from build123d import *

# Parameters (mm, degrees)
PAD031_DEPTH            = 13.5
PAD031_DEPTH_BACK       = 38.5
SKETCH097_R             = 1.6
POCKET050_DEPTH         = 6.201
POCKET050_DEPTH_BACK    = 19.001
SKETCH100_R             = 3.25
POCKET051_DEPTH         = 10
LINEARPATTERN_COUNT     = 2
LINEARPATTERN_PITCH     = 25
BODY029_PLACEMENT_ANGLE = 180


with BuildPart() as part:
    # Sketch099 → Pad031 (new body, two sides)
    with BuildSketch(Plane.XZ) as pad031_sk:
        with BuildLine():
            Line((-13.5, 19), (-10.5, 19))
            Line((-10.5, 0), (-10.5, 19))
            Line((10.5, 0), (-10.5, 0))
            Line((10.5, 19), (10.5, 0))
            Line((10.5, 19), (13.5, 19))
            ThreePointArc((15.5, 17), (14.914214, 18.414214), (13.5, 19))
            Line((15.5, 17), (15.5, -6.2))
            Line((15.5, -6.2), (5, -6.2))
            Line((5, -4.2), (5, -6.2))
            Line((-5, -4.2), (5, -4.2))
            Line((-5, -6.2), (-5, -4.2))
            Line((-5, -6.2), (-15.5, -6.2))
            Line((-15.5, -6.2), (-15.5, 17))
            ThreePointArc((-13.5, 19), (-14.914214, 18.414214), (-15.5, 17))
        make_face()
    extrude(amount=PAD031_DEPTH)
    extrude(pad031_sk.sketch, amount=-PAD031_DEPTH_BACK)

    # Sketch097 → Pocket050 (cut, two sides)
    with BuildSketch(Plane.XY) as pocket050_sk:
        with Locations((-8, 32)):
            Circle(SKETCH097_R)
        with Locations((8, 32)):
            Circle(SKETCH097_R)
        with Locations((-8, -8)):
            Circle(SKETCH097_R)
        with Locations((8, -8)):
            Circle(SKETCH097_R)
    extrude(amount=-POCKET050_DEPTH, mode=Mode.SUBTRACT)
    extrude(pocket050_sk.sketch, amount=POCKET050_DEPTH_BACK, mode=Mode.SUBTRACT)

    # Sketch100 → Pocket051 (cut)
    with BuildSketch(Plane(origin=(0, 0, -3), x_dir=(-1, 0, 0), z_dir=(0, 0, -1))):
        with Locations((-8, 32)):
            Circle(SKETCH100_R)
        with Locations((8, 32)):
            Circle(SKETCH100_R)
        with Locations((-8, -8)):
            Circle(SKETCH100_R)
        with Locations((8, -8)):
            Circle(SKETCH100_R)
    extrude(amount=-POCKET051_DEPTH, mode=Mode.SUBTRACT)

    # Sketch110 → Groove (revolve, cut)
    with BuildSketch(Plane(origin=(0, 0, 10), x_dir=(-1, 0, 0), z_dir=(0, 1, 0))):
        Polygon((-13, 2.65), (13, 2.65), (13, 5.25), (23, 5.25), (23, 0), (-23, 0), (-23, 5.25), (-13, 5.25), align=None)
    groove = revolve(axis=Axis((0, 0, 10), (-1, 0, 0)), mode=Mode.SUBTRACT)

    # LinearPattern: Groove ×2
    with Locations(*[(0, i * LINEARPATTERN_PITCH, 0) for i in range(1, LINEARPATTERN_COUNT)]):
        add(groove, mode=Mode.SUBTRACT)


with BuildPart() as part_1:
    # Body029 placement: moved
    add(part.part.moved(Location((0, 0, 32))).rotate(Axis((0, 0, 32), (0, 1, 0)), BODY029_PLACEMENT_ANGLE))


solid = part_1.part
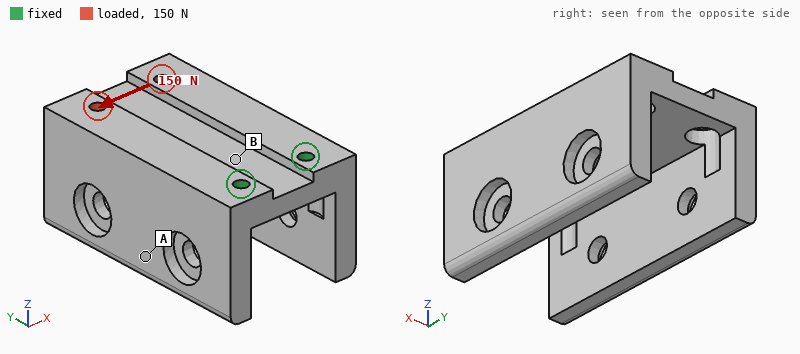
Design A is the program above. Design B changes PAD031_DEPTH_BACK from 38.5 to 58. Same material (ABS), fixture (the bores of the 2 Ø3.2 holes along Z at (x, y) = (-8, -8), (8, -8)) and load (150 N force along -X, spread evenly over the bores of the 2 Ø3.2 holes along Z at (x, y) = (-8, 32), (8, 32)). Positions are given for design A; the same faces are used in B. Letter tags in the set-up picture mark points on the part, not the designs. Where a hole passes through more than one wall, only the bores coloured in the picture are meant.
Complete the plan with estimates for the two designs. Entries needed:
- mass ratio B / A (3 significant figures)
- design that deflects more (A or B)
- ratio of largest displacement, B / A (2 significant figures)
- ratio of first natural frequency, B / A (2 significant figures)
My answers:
1.41
B
1.2
0.59
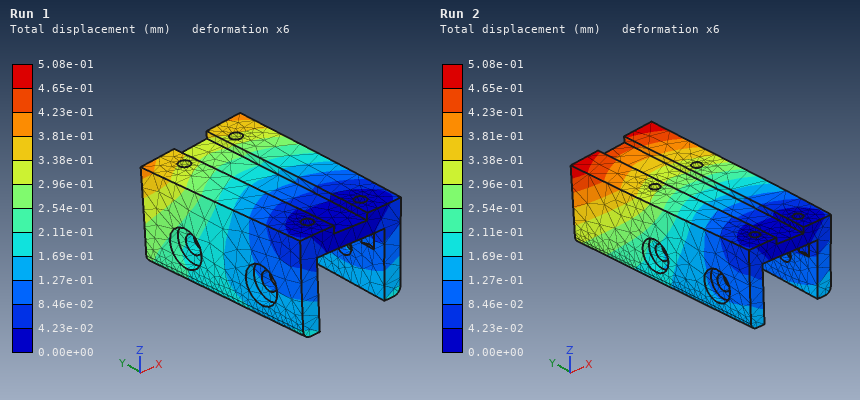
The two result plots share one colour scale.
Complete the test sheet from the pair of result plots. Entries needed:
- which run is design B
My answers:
Run 2
